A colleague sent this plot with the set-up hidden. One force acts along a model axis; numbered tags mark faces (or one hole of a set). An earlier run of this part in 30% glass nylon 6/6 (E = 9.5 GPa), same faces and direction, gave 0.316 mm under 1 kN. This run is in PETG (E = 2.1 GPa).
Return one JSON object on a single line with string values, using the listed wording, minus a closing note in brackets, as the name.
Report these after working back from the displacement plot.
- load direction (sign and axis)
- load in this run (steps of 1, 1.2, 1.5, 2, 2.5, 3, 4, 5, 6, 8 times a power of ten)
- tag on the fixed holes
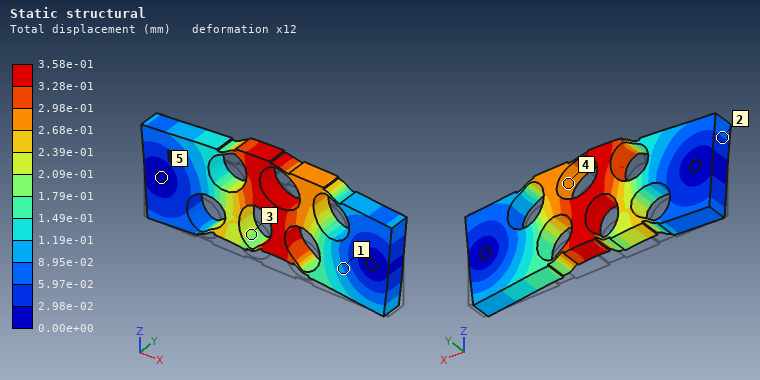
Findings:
{"load direction": "+Z", "load in this run": "250 N", "tag on the fixed holes": "5"}
